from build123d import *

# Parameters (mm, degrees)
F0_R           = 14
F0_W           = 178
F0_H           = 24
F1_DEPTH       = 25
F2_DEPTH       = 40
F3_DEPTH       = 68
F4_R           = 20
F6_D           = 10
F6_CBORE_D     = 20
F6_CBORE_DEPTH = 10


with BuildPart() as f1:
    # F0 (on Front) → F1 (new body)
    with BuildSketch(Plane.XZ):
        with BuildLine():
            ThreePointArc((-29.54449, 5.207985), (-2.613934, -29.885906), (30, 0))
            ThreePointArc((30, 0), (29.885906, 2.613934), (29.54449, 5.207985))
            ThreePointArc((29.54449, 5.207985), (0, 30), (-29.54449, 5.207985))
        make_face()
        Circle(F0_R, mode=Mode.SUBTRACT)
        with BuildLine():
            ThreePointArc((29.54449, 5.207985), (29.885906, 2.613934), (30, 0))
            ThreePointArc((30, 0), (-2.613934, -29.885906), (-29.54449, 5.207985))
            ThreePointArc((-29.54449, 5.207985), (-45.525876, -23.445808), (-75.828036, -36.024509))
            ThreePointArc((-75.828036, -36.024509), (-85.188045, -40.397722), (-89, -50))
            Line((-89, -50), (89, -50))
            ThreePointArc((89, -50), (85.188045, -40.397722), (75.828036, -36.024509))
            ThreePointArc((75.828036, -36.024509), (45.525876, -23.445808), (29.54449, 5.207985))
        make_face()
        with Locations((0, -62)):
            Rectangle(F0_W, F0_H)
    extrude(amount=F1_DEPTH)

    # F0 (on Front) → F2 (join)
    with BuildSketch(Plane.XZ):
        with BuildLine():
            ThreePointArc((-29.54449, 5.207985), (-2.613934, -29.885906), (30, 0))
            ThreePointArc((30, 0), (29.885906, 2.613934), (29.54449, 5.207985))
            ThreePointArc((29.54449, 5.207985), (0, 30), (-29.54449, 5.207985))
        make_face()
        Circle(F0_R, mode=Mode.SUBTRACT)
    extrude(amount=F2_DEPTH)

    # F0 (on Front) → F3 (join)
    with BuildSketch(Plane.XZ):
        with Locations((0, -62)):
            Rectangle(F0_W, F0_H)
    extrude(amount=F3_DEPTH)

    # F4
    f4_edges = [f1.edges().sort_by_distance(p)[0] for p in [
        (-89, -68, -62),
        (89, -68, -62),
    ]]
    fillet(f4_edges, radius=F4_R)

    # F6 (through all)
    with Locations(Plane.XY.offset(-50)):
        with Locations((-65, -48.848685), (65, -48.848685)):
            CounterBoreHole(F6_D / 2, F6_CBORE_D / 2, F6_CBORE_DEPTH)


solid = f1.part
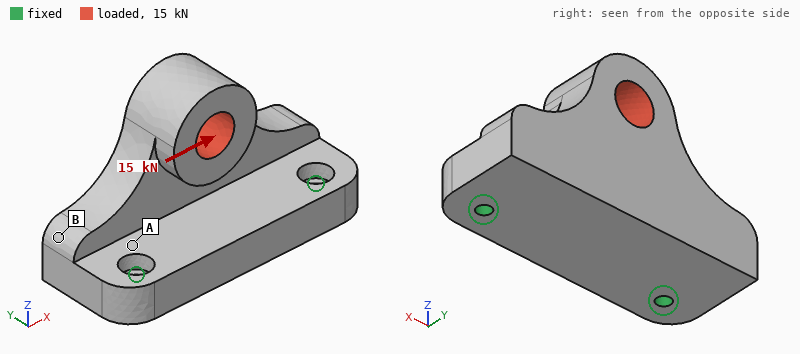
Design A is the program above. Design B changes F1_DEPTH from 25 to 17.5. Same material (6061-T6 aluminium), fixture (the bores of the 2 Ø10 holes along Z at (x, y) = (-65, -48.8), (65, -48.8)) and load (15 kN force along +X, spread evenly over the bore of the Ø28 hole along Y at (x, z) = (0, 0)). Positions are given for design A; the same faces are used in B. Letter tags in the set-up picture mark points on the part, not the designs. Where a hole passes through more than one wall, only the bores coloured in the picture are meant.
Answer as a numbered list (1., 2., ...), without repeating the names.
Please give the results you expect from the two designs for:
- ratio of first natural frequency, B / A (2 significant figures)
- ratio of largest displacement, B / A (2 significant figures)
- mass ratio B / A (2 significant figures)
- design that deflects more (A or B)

1. 0.95
2. 1.6
3. 0.93
4. B
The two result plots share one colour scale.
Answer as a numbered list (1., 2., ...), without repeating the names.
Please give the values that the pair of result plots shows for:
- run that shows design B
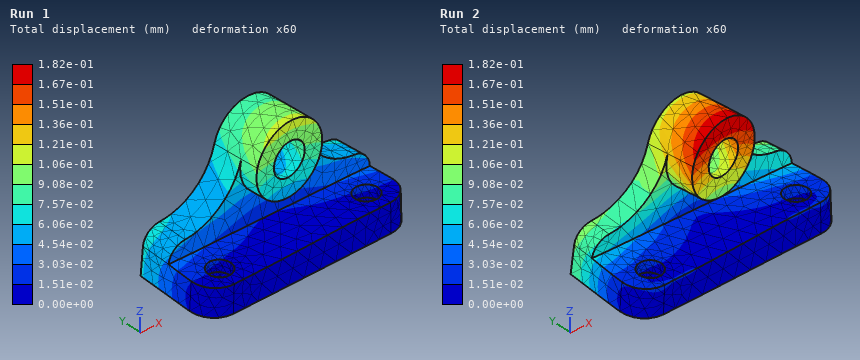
1. Run 2
